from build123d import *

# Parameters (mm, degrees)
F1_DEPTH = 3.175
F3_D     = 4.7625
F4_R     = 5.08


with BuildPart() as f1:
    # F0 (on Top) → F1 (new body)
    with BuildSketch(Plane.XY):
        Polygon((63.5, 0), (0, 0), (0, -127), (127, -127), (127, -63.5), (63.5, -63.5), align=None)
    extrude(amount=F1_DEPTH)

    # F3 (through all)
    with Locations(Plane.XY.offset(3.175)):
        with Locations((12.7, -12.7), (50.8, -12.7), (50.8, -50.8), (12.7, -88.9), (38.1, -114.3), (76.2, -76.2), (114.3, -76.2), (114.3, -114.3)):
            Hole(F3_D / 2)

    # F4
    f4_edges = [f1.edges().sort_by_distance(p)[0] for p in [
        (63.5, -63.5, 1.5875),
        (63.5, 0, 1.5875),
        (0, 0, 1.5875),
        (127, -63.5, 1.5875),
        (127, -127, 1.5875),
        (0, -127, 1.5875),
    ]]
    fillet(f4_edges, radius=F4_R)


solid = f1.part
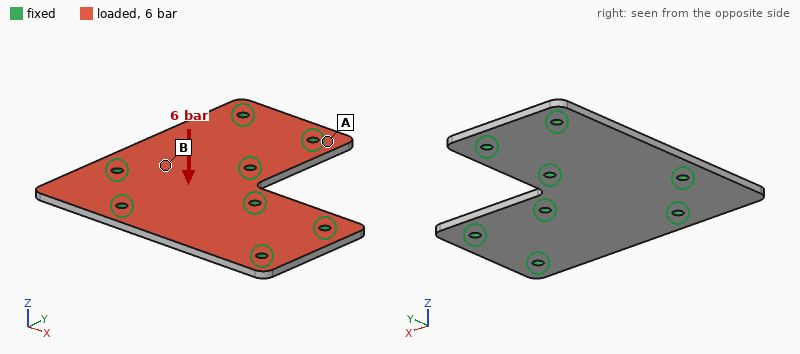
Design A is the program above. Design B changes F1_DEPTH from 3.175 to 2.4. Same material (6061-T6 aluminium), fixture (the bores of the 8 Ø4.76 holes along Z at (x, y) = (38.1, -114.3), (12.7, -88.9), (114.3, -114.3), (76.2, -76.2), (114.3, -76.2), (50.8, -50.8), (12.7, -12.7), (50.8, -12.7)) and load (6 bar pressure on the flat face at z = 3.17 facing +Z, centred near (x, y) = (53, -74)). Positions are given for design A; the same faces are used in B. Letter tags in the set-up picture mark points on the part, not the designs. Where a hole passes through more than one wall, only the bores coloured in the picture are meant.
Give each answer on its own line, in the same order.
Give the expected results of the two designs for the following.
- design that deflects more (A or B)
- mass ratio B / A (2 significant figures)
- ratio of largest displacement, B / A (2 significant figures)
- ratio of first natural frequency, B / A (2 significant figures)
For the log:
B
0.76
2.2
0.77
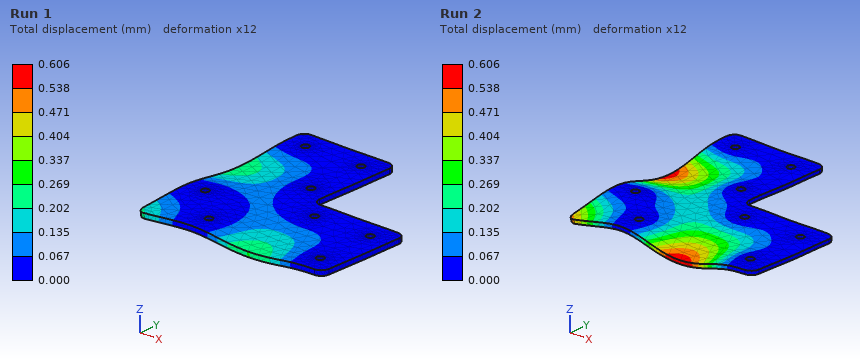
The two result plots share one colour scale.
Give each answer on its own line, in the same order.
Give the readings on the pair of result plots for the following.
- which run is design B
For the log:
Run 2
